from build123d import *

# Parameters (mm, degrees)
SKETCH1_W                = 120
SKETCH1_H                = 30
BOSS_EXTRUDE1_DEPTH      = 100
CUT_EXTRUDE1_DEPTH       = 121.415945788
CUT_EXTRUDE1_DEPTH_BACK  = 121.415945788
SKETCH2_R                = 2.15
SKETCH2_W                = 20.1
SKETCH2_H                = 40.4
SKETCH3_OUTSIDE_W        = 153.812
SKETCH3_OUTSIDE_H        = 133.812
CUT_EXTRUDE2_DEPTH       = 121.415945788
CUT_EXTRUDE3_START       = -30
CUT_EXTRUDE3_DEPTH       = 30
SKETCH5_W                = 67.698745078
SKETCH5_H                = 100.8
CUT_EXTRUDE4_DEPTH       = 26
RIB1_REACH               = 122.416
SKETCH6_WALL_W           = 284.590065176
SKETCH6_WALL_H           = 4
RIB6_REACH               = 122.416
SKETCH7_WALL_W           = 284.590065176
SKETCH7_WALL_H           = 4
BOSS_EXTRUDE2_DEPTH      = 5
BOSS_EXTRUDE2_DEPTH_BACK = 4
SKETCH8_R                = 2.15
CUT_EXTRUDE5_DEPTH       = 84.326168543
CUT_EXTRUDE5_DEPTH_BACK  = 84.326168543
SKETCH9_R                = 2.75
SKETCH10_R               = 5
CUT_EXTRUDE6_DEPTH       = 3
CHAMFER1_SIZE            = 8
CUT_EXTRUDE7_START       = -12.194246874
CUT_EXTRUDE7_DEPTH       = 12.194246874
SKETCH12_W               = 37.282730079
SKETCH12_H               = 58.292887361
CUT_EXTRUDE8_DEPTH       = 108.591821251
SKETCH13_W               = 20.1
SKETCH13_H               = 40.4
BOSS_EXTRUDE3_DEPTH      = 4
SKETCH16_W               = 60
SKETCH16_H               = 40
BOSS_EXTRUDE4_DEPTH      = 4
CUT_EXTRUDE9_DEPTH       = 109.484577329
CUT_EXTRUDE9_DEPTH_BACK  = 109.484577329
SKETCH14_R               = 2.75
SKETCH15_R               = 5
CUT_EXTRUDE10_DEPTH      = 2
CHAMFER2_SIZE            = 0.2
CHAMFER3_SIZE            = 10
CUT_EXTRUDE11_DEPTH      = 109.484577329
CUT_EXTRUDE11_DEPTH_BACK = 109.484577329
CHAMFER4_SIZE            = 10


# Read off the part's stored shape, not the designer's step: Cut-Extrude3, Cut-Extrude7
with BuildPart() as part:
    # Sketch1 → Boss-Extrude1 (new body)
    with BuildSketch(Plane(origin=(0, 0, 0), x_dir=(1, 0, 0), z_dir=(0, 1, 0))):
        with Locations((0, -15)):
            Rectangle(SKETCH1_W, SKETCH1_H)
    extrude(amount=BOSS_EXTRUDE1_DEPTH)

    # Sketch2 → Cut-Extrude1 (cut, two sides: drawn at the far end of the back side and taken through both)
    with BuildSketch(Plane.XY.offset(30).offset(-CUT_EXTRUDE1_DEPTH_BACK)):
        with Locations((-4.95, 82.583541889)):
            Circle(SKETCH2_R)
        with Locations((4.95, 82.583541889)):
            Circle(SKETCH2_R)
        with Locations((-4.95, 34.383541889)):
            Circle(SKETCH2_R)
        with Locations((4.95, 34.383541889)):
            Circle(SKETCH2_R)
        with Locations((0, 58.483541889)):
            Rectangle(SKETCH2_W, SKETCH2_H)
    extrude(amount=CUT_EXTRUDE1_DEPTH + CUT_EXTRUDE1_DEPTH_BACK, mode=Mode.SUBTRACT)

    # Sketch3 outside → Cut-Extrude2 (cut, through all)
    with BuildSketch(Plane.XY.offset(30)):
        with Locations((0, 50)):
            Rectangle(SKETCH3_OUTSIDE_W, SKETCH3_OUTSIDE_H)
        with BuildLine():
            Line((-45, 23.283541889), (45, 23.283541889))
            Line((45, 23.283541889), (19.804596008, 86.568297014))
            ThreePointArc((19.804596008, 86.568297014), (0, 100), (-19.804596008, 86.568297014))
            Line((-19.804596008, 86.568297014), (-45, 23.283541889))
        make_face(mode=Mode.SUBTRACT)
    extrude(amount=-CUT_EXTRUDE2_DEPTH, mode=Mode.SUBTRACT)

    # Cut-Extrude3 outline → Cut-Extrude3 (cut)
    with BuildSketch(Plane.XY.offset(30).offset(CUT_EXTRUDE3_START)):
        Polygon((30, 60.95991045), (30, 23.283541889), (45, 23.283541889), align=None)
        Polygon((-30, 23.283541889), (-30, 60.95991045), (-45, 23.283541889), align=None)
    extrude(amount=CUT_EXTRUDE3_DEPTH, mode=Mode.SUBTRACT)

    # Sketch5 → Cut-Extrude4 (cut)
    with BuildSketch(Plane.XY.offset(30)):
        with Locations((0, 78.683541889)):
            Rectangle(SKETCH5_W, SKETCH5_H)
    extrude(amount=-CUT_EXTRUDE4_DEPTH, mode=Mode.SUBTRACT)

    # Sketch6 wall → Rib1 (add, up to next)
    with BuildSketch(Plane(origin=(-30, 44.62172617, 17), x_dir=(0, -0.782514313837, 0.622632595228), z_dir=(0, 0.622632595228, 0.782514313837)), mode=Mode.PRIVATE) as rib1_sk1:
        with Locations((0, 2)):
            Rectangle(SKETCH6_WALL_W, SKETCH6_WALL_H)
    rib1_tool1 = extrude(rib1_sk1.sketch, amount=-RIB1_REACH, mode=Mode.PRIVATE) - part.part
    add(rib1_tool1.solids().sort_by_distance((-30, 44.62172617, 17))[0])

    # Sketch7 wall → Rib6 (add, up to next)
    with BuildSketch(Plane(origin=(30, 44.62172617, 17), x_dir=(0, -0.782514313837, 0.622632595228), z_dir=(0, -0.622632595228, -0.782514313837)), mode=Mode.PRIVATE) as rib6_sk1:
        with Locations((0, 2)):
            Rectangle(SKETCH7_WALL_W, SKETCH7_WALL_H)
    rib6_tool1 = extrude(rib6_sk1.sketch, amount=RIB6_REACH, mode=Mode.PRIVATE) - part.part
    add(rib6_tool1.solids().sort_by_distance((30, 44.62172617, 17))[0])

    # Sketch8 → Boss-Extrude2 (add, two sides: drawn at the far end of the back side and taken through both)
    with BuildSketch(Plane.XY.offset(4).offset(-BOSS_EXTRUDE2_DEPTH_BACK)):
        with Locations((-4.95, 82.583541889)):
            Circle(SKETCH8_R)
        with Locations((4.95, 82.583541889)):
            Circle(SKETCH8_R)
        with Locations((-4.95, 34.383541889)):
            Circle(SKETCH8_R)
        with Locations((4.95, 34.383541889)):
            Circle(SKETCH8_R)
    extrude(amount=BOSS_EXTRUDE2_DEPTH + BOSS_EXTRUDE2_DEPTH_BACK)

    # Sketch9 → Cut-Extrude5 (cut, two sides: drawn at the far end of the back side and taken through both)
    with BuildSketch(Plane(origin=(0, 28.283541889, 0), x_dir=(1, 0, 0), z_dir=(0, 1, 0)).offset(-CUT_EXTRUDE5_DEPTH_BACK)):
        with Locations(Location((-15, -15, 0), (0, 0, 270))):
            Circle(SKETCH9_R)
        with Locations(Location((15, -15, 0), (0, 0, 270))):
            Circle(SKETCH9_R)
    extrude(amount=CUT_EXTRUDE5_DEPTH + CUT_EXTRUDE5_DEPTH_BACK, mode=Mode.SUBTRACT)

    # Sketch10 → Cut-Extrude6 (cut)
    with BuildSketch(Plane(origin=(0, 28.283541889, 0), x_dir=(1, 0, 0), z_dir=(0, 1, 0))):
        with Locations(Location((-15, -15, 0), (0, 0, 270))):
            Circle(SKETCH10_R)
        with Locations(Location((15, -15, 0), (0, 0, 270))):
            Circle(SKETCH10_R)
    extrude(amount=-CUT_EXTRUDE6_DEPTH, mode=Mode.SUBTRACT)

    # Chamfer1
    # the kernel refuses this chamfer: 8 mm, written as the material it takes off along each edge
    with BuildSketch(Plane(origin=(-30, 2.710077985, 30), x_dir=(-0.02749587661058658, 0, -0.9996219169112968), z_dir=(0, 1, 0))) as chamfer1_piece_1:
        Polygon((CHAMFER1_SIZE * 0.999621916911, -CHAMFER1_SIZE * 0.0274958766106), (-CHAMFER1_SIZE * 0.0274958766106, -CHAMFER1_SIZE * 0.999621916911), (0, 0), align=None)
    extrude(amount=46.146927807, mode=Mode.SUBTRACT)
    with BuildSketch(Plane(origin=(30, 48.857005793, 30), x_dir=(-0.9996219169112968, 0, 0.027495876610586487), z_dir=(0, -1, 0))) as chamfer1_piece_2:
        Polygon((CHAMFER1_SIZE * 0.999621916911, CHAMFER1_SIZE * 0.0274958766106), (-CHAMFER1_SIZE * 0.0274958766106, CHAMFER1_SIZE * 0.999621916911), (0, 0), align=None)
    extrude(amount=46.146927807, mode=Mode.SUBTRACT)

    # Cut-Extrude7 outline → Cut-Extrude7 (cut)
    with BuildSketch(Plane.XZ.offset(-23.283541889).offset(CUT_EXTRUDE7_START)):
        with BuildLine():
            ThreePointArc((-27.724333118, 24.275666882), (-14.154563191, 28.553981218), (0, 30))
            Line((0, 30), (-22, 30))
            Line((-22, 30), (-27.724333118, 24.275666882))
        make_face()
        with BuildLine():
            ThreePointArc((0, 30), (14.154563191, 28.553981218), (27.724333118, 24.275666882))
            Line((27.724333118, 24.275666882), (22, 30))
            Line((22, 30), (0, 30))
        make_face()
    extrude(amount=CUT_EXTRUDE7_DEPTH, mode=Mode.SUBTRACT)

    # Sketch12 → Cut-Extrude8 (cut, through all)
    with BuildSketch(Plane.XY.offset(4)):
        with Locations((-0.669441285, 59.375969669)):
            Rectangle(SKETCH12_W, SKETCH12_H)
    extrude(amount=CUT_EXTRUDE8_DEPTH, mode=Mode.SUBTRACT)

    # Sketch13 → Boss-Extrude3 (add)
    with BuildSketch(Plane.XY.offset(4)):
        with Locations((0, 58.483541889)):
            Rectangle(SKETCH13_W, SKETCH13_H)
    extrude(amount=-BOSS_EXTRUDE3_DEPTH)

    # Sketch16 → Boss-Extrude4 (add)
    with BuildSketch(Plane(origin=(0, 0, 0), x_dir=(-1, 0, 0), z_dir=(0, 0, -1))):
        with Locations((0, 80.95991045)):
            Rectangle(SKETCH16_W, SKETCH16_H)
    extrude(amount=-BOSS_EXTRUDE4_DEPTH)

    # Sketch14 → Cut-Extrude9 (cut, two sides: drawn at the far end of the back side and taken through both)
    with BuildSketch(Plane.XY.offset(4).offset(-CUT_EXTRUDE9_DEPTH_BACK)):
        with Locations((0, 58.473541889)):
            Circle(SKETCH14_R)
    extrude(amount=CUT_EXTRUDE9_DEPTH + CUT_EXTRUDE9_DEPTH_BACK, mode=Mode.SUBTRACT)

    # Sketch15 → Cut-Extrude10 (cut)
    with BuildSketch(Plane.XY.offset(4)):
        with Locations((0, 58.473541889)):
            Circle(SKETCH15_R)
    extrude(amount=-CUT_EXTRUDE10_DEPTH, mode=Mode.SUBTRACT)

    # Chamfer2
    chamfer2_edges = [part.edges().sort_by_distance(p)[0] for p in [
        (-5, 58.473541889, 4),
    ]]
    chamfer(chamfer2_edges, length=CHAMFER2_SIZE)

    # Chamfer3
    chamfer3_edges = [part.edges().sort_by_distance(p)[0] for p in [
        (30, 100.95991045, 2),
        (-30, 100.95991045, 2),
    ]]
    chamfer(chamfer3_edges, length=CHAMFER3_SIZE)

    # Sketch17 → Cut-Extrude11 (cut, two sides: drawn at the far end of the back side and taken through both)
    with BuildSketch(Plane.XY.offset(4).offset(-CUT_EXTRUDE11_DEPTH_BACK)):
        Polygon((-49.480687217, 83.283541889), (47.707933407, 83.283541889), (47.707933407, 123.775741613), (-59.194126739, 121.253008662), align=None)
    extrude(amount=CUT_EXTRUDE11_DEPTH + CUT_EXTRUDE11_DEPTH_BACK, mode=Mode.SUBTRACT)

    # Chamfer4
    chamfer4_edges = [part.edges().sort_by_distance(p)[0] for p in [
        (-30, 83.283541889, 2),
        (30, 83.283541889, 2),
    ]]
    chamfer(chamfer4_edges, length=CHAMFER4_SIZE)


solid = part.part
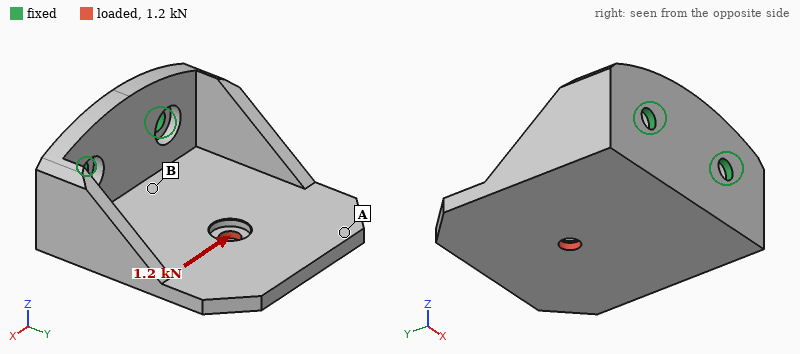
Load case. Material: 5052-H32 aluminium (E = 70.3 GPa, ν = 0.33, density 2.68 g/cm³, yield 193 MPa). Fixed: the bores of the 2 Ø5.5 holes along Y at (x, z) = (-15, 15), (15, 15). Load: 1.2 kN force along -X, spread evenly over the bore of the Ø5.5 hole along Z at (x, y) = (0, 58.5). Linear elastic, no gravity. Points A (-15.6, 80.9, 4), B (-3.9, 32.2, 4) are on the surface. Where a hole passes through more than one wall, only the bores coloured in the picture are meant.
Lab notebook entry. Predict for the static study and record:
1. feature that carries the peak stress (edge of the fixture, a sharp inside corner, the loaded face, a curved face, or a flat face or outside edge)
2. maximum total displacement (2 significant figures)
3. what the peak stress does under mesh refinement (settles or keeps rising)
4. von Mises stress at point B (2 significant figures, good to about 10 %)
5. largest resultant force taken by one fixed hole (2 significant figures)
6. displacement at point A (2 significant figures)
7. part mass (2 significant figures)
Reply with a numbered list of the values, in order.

1. edge of the fixture
2. 0.21 mm
3. keeps rising
4. 42 MPa
5. 1.5 kN
6. 0.18 mm
7. 63 g
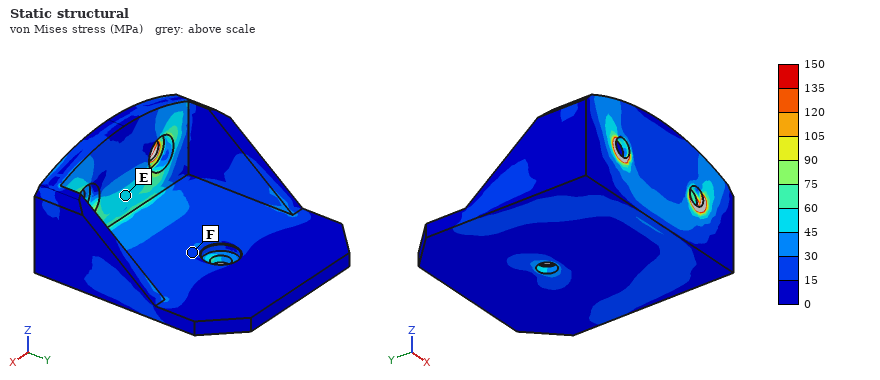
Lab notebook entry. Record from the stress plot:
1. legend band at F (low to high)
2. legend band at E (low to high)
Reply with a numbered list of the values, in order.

1. 15 to 30 MPa
2. 45 to 60 MPa
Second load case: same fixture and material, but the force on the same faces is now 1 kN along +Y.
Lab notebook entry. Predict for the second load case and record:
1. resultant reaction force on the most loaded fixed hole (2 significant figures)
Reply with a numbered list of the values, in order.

1. 510 N
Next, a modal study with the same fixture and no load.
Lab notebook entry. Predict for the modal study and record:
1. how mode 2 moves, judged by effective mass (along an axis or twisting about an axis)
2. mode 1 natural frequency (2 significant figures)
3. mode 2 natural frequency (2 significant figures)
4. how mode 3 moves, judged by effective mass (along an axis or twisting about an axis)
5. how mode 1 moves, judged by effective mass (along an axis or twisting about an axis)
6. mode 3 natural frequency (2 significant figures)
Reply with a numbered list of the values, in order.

1. along X
2. 1000 Hz
3. 2100 Hz
4. along X
5. along Z
6. 4300 Hz
